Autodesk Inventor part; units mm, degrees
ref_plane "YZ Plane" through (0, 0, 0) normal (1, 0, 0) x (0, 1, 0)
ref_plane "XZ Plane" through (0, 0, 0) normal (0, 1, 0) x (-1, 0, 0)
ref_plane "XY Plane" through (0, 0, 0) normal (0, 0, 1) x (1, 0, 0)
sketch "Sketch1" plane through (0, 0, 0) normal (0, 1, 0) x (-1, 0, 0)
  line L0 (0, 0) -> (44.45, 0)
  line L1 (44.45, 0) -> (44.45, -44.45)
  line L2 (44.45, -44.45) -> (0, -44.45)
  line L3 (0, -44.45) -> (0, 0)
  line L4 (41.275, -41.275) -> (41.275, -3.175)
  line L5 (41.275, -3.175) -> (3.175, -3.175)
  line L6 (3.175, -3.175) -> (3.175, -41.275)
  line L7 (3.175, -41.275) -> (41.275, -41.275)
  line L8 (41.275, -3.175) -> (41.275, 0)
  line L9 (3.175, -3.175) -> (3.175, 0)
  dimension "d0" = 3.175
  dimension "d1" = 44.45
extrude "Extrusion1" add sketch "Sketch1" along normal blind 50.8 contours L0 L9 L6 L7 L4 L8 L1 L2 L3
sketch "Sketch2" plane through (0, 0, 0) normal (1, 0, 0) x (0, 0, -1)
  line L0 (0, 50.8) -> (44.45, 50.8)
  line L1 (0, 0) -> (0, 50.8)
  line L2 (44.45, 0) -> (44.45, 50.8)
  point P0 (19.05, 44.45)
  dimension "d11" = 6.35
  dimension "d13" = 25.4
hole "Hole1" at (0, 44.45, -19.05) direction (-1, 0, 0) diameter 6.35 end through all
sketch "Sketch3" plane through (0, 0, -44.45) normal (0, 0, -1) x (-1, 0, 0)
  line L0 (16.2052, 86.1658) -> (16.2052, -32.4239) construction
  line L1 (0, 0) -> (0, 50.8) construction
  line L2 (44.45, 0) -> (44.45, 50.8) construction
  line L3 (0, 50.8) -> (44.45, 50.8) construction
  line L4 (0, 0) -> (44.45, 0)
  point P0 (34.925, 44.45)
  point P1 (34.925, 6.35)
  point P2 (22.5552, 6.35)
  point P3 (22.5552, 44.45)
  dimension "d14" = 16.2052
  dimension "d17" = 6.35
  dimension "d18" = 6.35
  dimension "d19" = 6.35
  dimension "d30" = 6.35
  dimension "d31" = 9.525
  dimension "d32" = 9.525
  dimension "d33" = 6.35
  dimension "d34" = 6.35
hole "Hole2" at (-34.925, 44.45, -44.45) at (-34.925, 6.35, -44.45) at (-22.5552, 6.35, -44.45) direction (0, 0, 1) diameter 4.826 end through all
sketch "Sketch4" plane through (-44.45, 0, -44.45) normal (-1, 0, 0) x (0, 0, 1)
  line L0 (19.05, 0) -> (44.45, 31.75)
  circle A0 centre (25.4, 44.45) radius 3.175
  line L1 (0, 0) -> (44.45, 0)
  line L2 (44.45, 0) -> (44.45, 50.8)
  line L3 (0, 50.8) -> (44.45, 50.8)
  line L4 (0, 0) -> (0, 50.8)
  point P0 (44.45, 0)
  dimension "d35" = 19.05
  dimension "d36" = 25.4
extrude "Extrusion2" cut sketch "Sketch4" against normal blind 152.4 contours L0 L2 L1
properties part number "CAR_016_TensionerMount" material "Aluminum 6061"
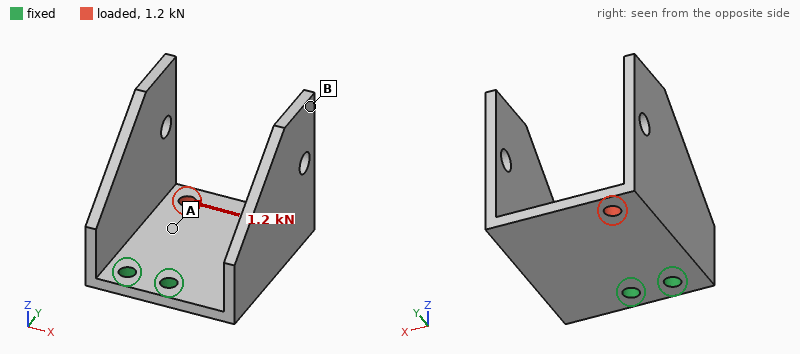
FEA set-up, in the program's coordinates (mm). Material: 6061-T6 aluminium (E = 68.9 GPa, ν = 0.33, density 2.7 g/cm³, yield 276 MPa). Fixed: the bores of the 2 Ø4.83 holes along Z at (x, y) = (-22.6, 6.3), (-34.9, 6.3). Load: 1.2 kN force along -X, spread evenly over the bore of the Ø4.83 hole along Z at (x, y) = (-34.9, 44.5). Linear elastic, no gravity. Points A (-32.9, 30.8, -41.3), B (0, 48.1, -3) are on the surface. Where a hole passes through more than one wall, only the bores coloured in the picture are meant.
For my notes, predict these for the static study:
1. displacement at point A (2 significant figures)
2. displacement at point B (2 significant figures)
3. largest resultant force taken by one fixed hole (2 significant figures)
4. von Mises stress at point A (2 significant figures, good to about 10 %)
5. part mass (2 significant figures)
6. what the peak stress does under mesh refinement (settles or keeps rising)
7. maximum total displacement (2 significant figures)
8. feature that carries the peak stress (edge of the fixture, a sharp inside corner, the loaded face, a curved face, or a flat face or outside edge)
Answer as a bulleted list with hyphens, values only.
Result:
- 0.044 mm
- 0.096 mm
- 2.7 kN
- 25 MPa
- 47 g
- keeps rising
- 0.10 mm
- edge of the fixture
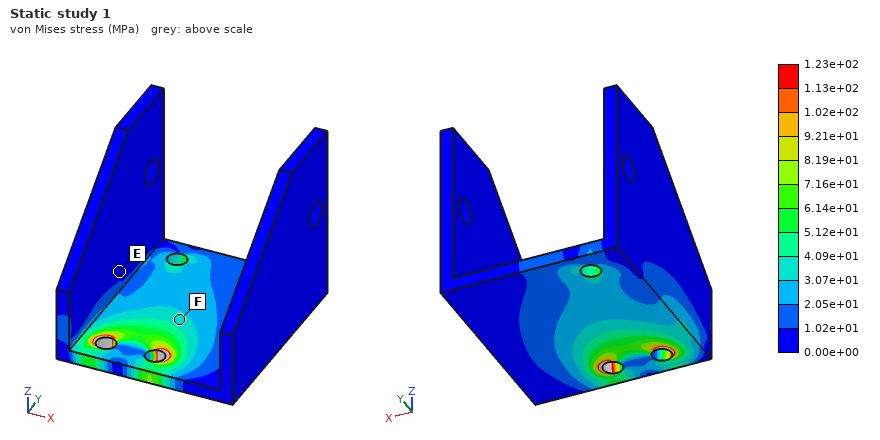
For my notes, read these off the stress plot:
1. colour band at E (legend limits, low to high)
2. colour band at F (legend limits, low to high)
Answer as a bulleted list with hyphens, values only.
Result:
- 0.00e+00 to 1.02e+01 MPa
- 3.07e+01 to 4.09e+01 MPa
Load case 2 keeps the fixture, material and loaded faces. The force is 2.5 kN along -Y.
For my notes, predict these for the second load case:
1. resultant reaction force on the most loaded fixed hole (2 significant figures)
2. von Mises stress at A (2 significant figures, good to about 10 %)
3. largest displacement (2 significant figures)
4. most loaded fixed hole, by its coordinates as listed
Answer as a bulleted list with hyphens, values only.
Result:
- 2.2 kN
- 33 MPa
- 38 µm
- (-34.9, 6.3)
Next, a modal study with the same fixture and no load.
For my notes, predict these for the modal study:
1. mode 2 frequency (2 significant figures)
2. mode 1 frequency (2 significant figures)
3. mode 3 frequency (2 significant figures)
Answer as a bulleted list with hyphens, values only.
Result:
- 1000 Hz
- 730 Hz
- 1200 Hz
